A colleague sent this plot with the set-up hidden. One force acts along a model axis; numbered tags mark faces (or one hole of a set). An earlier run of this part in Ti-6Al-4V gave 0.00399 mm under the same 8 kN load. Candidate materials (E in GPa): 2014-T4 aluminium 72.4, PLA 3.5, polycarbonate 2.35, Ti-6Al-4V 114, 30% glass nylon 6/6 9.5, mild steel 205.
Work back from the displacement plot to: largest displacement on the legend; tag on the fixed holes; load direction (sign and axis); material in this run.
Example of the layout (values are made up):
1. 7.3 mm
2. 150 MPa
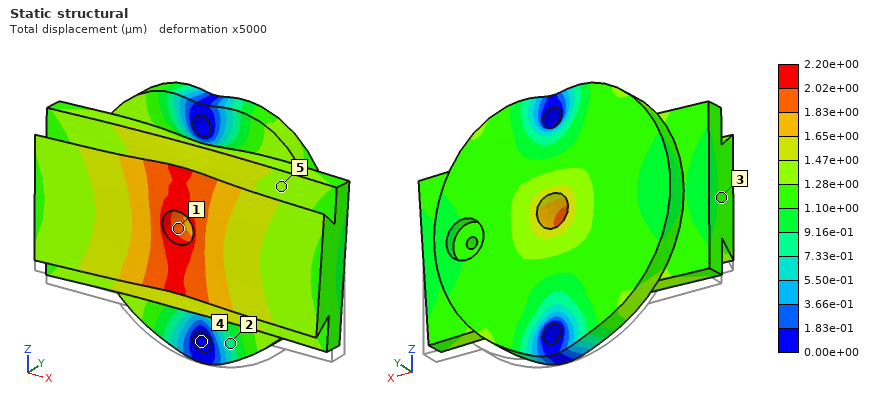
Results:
1. 2.20e+00 µm
2. 4
3. +Z
4. mild steel
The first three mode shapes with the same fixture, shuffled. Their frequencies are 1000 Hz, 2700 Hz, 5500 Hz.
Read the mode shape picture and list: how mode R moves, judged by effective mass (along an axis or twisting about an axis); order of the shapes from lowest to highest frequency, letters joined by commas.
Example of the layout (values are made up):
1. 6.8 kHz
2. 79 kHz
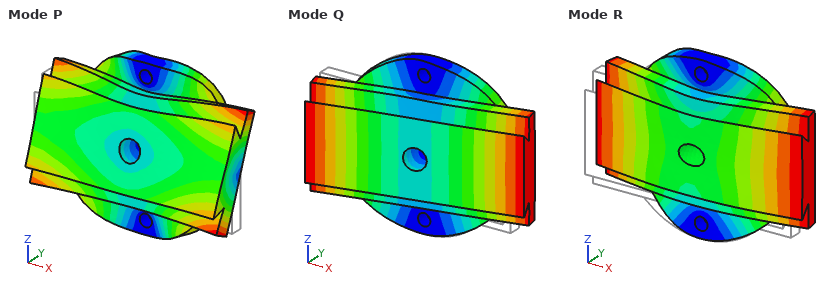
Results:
1. along Y
2. Q, R, P
